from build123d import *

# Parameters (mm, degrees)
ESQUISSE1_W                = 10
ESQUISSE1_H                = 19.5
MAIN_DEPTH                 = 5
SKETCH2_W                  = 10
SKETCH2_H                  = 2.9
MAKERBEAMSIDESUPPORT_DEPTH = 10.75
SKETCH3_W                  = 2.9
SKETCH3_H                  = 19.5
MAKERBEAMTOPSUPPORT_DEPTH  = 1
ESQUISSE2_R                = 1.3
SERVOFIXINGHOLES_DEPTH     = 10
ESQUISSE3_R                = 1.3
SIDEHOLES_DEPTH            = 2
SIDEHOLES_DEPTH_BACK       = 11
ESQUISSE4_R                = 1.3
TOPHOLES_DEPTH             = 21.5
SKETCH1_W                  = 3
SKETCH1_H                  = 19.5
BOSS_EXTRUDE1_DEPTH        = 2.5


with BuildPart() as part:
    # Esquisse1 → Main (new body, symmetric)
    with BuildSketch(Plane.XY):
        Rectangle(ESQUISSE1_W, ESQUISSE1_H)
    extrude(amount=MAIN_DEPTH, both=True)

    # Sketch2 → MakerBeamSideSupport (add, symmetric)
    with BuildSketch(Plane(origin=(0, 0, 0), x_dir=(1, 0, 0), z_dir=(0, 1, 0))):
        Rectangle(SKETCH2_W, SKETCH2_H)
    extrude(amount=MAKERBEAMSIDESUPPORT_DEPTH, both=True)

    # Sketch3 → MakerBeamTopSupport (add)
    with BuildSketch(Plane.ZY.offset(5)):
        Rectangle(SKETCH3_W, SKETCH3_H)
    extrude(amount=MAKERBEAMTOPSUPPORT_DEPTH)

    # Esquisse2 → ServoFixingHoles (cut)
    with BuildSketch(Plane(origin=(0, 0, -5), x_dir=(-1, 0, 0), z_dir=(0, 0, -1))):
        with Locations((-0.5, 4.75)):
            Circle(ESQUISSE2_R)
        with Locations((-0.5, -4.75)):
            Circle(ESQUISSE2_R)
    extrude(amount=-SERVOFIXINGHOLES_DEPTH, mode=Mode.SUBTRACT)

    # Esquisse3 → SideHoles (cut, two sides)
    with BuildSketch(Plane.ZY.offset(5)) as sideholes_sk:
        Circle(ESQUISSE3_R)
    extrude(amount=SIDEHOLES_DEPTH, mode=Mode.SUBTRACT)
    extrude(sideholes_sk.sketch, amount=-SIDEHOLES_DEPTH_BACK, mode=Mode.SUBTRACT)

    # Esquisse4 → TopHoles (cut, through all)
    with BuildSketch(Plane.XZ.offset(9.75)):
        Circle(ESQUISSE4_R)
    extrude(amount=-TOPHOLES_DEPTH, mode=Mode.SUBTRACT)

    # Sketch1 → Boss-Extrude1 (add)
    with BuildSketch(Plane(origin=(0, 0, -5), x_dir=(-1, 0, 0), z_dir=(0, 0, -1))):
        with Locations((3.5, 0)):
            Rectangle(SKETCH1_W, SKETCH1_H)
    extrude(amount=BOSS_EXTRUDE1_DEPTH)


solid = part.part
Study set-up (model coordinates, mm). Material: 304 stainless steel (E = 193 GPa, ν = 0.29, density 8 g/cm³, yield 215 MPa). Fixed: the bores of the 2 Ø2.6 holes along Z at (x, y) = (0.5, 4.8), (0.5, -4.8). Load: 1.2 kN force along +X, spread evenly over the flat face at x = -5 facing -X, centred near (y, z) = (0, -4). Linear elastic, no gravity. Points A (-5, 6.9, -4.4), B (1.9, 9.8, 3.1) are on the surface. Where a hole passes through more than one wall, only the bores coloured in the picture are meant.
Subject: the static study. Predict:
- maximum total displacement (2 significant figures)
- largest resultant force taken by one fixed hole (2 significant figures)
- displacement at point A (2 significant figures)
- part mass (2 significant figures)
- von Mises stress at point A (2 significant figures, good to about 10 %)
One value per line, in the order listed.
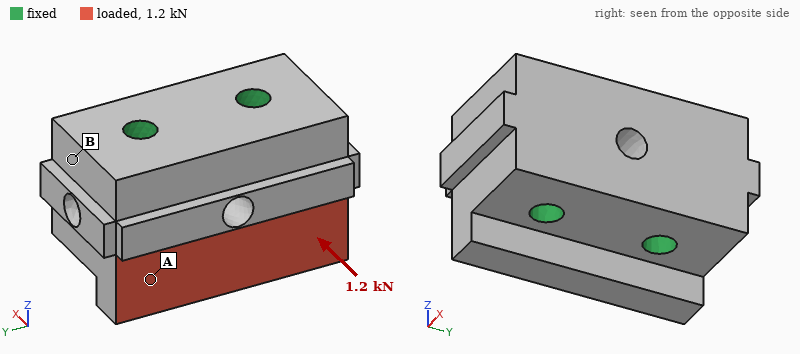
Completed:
1.9 µm
600 N
0.97 µm
16 g
25 MPa
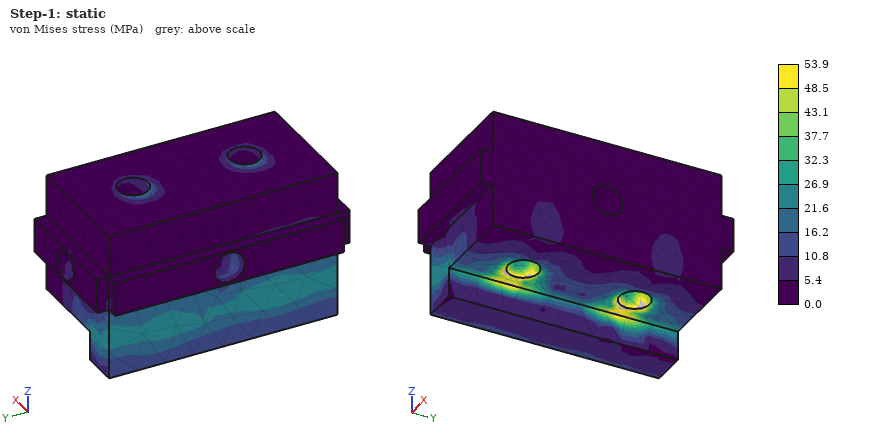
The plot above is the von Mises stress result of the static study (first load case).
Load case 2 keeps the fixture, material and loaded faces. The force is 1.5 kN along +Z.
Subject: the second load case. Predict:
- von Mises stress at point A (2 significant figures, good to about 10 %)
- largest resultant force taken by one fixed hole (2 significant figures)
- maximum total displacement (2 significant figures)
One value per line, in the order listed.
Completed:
47 MPa
750 N
3.4 µm
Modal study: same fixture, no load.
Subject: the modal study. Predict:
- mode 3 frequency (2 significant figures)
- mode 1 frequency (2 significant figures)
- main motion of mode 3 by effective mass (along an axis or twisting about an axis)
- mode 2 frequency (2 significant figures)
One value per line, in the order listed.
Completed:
84 kHz
74 kHz
twisting about X
77 kHz
